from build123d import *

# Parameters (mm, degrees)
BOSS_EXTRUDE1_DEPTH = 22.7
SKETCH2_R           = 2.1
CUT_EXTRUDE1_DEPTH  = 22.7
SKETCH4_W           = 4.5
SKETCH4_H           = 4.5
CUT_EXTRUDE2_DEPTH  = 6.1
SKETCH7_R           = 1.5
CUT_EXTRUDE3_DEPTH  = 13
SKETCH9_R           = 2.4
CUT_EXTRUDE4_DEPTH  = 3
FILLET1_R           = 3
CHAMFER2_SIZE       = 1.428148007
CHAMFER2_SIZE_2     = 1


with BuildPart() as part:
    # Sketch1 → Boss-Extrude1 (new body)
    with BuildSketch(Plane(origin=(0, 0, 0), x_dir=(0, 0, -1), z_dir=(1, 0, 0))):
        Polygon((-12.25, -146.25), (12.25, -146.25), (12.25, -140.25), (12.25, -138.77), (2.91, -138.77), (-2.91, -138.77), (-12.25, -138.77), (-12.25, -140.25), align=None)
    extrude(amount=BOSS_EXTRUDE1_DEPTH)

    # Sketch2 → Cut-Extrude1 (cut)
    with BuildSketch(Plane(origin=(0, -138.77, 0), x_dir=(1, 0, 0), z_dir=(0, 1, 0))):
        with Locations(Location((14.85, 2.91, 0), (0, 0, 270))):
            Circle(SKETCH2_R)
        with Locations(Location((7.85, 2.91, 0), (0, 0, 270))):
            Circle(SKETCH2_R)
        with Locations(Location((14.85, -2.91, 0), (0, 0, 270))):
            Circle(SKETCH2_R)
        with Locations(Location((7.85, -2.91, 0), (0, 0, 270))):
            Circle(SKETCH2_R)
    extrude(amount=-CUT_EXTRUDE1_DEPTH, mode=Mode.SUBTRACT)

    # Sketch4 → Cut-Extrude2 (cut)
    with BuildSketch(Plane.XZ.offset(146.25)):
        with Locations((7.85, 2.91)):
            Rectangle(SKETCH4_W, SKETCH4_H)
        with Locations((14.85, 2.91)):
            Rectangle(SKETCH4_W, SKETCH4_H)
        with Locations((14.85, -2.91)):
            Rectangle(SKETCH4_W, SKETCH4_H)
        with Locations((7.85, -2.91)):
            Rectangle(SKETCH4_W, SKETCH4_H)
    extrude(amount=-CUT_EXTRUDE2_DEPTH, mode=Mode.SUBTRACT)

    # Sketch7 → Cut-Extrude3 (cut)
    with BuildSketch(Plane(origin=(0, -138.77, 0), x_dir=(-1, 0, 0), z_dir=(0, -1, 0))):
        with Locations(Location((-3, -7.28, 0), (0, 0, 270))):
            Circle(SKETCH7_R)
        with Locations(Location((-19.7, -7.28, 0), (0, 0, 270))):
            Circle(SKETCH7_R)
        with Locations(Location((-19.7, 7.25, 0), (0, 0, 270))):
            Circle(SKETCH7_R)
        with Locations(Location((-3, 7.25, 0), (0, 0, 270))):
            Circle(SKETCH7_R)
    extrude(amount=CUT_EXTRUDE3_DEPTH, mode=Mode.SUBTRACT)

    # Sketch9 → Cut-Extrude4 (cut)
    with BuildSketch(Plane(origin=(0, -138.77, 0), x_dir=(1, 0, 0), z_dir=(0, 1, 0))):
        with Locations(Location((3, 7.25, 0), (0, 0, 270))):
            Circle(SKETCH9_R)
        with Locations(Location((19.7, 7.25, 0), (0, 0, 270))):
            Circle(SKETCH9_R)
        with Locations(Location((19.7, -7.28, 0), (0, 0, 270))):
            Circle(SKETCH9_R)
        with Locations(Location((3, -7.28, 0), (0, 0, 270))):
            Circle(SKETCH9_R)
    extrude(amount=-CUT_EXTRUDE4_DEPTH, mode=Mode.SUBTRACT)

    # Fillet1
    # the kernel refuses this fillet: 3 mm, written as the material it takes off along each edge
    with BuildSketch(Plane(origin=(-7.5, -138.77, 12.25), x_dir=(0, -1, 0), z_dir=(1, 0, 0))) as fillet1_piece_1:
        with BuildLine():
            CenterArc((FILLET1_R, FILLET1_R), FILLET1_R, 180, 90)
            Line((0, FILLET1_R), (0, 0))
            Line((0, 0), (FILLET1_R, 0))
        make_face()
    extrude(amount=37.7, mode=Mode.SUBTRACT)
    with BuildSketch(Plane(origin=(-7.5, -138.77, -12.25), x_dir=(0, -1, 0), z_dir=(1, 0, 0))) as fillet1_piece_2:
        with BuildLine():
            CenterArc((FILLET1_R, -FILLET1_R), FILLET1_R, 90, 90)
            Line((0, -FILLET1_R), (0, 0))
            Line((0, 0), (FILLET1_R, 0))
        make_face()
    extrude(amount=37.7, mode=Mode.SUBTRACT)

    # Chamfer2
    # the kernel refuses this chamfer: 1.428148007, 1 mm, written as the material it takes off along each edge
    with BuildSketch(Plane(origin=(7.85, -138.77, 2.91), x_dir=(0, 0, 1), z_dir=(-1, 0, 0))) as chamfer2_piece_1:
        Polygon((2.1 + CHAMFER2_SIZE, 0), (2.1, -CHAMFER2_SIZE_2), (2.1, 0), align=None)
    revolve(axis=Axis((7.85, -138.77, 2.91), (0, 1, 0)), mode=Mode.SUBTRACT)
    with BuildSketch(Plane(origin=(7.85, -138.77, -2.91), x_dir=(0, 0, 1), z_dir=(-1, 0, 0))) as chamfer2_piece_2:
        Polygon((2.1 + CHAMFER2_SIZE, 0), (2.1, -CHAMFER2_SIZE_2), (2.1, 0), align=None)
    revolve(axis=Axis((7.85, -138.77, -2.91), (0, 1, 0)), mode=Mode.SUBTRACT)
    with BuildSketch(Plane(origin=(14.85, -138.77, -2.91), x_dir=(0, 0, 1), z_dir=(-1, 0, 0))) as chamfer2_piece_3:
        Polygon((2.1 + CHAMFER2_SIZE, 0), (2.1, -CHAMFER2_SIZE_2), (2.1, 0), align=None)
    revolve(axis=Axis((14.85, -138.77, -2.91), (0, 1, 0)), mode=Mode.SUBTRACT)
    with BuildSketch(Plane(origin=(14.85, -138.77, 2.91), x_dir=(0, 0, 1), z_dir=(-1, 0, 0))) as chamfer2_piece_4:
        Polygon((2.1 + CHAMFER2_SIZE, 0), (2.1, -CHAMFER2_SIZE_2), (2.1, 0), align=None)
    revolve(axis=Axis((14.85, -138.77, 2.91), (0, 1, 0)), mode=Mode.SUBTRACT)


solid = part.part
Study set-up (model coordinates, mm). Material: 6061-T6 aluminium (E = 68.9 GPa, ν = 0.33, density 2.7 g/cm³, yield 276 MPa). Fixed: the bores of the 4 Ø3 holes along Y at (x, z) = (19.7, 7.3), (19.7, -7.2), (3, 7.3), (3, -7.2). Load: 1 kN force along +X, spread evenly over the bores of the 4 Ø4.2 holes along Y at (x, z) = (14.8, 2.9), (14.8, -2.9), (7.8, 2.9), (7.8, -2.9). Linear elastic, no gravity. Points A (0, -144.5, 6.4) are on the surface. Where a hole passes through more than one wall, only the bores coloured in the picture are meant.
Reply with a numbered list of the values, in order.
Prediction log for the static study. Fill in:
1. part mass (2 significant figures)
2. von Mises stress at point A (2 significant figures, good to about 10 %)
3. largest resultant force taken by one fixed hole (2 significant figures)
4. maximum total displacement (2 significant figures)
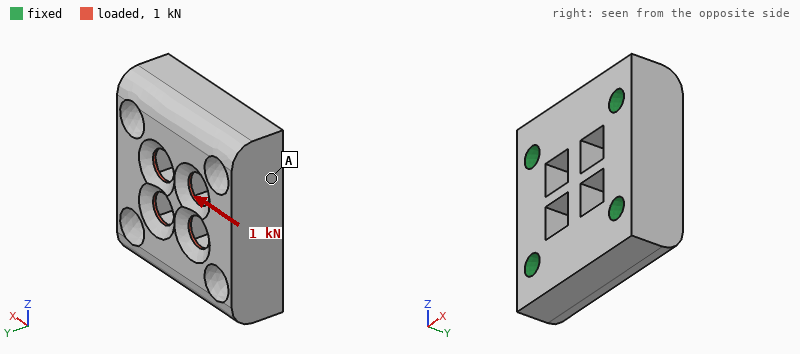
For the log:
1. 8.4 g
2. 8.1 MPa
3. 280 N
4. 3.7 µm
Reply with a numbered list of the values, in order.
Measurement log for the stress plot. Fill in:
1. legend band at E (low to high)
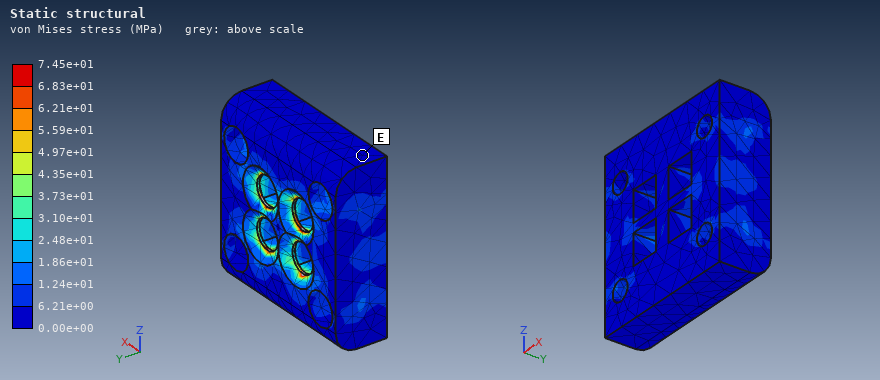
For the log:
1. 0.00e+00 to 6.21e+00 MPa
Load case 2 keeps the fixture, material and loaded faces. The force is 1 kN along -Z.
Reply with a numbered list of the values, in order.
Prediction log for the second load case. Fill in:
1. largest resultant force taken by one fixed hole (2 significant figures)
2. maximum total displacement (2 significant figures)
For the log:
1. 270 N
2. 4.5 µm
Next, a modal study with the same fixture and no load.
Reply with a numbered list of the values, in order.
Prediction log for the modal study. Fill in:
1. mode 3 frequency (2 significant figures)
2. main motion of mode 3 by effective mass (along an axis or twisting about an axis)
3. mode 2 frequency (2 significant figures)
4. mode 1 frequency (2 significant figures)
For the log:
1. 66 kHz
2. along Z
3. 59 kHz
4. 57 kHz
